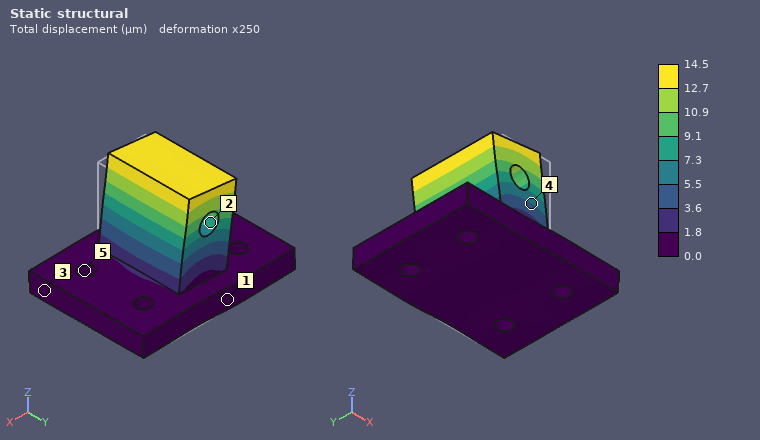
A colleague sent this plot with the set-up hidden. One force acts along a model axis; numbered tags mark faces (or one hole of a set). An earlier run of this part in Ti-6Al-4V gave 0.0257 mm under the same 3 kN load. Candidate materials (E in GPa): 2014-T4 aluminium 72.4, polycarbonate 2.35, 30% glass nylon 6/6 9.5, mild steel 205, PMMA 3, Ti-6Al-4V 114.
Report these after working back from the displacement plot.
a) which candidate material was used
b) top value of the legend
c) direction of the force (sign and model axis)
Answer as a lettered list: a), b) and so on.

a) mild steel
b) 14.5 µm
c) -X
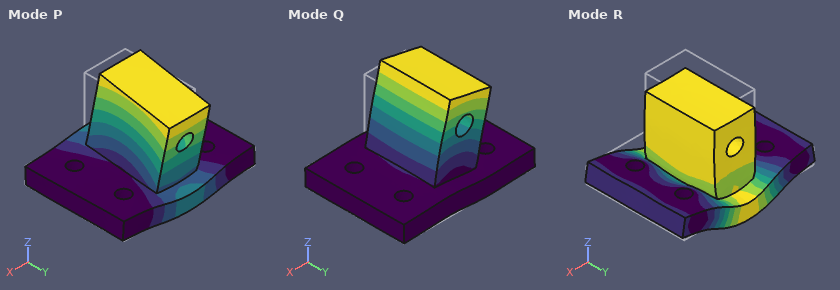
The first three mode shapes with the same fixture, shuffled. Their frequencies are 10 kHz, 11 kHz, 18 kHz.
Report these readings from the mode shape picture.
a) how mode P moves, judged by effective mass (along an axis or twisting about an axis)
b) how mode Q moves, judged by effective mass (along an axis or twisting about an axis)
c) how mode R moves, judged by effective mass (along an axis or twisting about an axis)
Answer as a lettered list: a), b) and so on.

a) along Y
b) along X
c) along Z
